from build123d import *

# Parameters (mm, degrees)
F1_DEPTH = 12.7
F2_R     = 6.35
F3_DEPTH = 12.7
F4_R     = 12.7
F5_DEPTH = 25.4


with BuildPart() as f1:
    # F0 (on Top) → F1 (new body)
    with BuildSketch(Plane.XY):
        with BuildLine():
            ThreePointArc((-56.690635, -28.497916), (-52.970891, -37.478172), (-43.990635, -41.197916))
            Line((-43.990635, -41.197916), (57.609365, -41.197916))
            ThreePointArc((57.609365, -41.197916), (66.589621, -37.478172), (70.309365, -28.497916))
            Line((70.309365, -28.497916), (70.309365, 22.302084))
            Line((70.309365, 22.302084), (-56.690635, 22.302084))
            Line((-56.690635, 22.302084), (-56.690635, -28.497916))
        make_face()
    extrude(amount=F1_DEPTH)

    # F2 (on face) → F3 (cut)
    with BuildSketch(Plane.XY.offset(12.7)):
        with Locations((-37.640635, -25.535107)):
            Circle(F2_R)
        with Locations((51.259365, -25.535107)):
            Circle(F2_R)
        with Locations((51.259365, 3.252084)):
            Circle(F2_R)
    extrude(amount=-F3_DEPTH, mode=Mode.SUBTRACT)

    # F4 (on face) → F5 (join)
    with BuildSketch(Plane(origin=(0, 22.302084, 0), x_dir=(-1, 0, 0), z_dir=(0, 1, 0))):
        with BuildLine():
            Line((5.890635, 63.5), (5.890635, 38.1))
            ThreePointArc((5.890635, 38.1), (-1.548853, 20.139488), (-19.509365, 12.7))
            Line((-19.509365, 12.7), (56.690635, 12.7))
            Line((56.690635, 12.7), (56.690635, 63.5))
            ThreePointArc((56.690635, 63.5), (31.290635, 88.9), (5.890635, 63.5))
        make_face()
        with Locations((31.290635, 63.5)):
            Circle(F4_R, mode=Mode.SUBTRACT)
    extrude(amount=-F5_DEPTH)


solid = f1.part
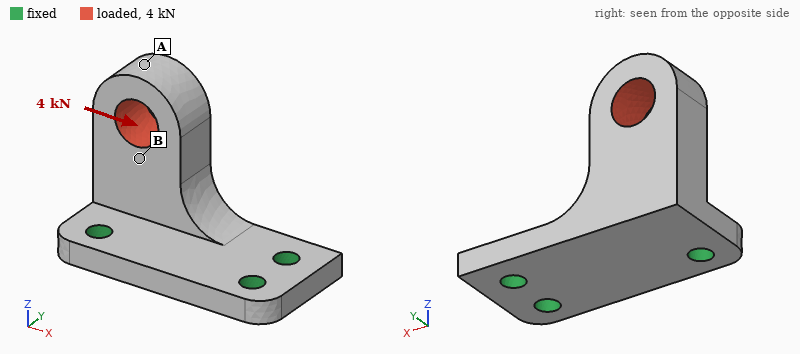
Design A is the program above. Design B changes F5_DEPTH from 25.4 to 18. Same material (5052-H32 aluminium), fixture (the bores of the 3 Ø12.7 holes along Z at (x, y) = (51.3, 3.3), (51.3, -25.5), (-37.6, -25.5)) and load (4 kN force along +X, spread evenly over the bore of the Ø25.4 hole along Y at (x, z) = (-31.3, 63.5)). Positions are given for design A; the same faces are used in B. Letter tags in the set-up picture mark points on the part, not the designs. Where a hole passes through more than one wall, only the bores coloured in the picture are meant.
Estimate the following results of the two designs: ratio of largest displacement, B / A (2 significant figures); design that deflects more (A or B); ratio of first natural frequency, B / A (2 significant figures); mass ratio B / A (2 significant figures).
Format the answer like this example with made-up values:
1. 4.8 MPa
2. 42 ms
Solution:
1. 1.4
2. B
3. 1.00
4. 0.87
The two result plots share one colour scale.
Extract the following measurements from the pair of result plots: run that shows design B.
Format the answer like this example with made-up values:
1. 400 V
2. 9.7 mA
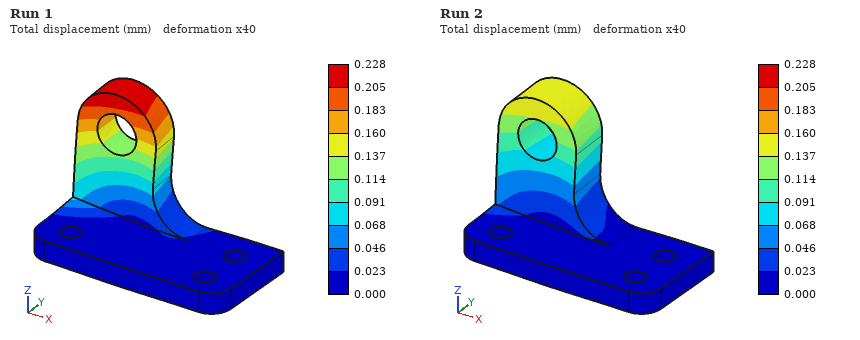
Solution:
1. Run 1
